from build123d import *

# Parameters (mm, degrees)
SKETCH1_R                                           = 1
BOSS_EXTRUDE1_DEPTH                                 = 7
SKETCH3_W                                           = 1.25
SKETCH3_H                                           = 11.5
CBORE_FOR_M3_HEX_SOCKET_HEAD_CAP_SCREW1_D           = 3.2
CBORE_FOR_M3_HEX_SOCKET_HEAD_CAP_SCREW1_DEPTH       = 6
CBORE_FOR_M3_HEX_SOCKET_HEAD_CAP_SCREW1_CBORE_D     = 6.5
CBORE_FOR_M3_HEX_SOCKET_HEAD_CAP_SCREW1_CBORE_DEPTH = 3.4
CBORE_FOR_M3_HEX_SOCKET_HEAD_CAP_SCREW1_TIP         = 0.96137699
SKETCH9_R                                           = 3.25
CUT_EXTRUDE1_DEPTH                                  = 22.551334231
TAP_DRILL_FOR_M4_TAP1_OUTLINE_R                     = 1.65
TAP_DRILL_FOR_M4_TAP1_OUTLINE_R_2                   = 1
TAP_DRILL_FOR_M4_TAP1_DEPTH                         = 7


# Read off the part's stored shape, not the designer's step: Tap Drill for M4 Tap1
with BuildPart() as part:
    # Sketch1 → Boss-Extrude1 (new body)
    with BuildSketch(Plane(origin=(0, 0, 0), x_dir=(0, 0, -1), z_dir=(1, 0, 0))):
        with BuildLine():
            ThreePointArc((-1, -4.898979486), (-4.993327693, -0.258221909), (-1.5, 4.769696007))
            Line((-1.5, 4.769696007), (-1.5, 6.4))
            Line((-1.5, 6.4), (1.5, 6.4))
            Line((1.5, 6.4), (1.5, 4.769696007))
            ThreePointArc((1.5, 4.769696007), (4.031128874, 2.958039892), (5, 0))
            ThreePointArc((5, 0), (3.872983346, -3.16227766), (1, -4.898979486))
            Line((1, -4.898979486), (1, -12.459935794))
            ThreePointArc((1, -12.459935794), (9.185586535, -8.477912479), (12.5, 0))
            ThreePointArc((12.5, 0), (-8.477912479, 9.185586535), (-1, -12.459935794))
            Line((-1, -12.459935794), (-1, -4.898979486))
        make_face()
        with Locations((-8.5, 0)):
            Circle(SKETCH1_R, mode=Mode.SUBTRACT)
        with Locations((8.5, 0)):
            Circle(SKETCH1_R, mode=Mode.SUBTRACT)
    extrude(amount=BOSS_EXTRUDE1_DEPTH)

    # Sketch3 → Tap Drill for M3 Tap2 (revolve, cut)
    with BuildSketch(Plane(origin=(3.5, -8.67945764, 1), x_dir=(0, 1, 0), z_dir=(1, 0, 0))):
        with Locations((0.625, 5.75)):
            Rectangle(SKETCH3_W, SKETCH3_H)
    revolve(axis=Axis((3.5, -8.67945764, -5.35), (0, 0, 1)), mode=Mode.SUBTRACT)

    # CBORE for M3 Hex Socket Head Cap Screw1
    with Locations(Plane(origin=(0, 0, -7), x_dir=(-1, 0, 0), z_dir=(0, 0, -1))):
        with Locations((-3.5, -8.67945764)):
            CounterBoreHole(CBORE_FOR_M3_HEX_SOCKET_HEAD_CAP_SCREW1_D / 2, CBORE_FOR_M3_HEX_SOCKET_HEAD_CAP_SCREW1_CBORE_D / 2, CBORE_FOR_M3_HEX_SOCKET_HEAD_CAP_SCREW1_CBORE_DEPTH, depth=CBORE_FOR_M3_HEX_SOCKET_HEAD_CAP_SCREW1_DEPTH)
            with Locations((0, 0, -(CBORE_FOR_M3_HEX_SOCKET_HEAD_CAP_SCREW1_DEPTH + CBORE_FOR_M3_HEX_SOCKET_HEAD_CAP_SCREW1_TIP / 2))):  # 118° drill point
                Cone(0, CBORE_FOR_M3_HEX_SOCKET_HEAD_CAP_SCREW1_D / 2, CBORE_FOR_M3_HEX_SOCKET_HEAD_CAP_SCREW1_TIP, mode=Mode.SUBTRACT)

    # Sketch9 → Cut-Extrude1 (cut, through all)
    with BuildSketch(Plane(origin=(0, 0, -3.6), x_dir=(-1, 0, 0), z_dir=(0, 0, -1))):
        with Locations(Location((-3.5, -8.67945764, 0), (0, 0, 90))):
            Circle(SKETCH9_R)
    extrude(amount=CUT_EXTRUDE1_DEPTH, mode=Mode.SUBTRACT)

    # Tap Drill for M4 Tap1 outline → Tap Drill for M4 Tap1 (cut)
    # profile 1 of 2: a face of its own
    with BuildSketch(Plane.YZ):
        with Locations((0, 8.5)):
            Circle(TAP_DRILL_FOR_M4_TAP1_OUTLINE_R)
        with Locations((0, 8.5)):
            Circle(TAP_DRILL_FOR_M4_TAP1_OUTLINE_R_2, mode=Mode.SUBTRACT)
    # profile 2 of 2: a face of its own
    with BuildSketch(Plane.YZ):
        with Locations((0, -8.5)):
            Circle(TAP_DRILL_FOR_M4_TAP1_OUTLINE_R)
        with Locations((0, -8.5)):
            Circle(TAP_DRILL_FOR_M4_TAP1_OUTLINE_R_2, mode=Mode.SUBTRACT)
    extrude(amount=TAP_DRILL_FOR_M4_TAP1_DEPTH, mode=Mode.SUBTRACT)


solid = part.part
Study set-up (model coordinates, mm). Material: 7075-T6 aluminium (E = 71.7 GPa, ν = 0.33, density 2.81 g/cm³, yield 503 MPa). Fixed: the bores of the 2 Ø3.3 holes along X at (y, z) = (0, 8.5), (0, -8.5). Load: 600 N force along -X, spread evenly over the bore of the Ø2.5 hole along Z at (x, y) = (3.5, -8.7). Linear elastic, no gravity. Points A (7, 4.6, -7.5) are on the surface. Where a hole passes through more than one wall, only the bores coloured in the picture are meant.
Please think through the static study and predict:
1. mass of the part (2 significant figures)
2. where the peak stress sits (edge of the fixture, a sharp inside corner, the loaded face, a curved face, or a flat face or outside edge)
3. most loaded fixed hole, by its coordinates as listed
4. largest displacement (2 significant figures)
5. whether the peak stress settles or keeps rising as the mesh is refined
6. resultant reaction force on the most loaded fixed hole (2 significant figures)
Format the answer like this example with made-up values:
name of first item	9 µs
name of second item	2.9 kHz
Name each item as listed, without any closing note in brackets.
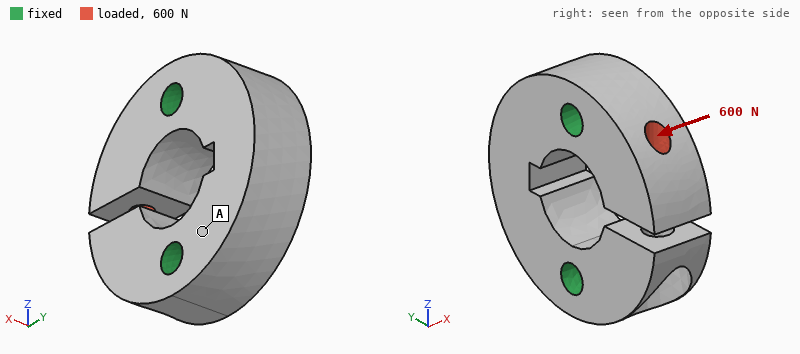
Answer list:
mass of the part	6.7 g
where the peak stress sits	edge of the fixture
most loaded fixed hole, by its coordinates as listed	(0, 8.5)
largest displacement	22 µm
whether the peak stress settles or keeps rising as the mesh is refined	keeps rising
resultant reaction force on the most loaded fixed hole	600 N
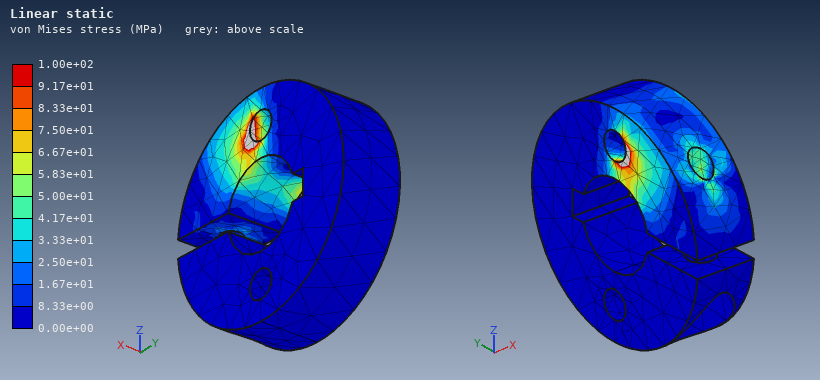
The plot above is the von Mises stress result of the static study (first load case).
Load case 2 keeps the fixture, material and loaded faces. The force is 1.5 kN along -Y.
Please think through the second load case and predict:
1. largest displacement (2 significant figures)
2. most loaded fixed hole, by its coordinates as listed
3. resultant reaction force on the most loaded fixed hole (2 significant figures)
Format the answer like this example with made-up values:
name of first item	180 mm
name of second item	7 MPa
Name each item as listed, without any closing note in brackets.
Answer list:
largest displacement	29 µm
most loaded fixed hole, by its coordinates as listed	(0, 8.5)
resultant reaction force on the most loaded fixed hole	1.4 kN
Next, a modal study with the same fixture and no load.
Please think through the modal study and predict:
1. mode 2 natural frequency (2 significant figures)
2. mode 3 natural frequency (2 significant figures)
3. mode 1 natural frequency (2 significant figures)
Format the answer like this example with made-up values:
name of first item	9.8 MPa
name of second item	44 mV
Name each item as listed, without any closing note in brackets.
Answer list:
mode 2 natural frequency	30 kHz
mode 3 natural frequency	31 kHz
mode 1 natural frequency	29 kHz
